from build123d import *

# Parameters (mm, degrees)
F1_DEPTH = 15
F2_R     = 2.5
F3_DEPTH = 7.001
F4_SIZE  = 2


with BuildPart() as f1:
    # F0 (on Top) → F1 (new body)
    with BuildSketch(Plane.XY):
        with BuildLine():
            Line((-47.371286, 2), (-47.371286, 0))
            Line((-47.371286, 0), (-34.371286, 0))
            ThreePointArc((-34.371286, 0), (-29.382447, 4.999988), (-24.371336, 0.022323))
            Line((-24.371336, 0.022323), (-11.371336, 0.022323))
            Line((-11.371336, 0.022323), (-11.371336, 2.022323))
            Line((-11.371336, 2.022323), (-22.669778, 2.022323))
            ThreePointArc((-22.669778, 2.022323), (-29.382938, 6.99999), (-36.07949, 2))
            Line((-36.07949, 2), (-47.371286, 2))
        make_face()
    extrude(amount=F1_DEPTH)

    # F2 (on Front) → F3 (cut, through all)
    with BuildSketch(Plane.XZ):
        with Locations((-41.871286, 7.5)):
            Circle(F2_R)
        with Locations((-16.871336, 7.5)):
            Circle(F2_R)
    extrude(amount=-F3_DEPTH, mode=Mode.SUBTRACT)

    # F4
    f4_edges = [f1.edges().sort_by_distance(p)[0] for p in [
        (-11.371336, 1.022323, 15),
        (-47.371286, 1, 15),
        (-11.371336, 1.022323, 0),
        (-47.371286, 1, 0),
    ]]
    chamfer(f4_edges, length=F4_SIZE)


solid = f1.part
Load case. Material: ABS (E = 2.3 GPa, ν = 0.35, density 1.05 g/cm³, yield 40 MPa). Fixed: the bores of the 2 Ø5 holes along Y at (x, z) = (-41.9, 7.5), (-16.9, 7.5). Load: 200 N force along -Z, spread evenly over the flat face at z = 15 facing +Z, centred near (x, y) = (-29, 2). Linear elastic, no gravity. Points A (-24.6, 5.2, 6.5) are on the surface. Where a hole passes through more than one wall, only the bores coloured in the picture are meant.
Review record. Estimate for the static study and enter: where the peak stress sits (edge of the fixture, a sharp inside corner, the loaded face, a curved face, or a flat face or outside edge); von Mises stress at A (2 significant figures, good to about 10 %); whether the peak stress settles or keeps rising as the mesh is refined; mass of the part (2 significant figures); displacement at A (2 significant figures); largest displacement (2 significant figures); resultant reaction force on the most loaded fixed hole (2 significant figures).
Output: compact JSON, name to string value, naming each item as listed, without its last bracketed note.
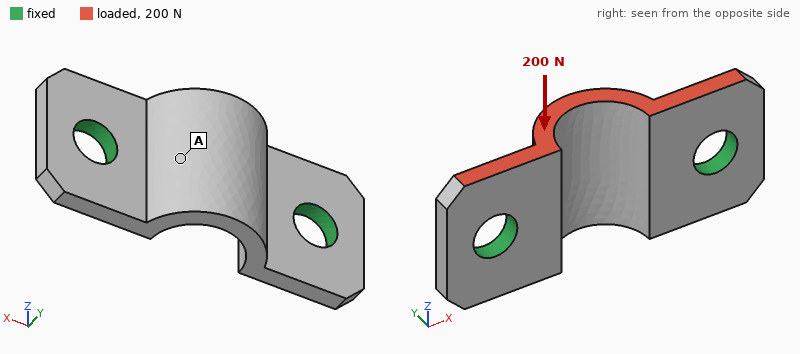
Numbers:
{"where the peak stress sits": "edge of the fixture", "von Mises stress at A": "3.9 MPa", "whether the peak stress settles or keeps rising as the mesh is refined": "keeps rising", "mass of the part": "1.2 g", "displacement at A": "0.097 mm", "largest displacement": "0.19 mm", "resultant reaction force on the most loaded fixed hole": "100 N"}
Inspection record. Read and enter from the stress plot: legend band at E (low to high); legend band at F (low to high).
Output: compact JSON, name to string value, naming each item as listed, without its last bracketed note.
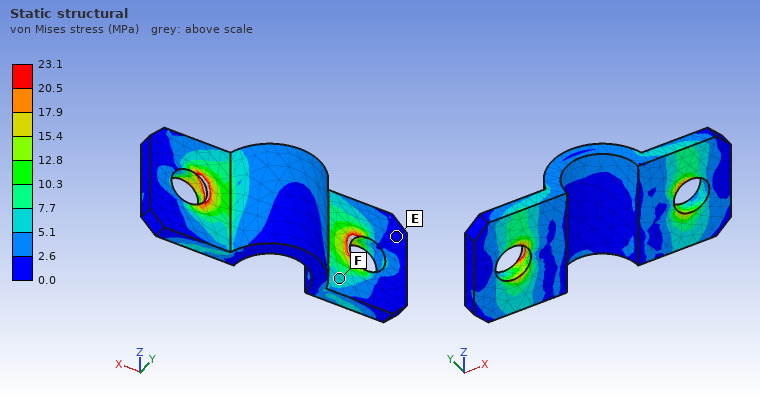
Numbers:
{"legend band at E": "0.0 to 2.6 MPa", "legend band at F": "5.1 to 7.7 MPa"}
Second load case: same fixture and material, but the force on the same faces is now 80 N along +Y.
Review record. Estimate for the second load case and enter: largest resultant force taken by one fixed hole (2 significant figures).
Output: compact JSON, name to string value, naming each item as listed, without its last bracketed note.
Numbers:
{"largest resultant force taken by one fixed hole": "44 N"}
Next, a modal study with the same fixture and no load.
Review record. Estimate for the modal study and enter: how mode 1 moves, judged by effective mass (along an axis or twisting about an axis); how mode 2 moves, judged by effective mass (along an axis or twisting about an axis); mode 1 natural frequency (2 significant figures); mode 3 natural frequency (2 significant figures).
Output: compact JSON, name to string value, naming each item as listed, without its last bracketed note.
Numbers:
{"how mode 1 moves, judged by effective mass": "along Z", "how mode 2 moves, judged by effective mass": "along Y", "mode 1 natural frequency": "5000 Hz", "mode 3 natural frequency": "11 kHz"}
